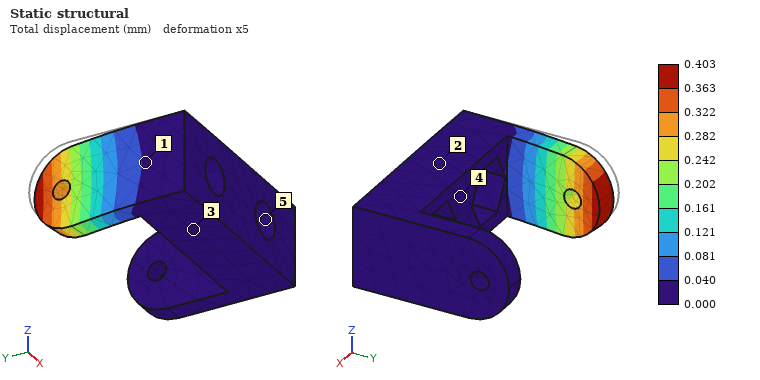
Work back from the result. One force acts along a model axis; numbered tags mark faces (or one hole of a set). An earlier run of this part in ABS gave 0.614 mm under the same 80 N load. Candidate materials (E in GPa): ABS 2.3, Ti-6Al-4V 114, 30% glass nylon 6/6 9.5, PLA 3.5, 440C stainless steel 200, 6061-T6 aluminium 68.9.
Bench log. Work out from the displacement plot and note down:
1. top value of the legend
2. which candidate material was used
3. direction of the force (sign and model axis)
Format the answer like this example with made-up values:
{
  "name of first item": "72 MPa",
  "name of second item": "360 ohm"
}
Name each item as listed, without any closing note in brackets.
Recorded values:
{
  "top value of the legend": "0.403 mm",
  "which candidate material was used": "PLA",
  "direction of the force": "+X"
}
